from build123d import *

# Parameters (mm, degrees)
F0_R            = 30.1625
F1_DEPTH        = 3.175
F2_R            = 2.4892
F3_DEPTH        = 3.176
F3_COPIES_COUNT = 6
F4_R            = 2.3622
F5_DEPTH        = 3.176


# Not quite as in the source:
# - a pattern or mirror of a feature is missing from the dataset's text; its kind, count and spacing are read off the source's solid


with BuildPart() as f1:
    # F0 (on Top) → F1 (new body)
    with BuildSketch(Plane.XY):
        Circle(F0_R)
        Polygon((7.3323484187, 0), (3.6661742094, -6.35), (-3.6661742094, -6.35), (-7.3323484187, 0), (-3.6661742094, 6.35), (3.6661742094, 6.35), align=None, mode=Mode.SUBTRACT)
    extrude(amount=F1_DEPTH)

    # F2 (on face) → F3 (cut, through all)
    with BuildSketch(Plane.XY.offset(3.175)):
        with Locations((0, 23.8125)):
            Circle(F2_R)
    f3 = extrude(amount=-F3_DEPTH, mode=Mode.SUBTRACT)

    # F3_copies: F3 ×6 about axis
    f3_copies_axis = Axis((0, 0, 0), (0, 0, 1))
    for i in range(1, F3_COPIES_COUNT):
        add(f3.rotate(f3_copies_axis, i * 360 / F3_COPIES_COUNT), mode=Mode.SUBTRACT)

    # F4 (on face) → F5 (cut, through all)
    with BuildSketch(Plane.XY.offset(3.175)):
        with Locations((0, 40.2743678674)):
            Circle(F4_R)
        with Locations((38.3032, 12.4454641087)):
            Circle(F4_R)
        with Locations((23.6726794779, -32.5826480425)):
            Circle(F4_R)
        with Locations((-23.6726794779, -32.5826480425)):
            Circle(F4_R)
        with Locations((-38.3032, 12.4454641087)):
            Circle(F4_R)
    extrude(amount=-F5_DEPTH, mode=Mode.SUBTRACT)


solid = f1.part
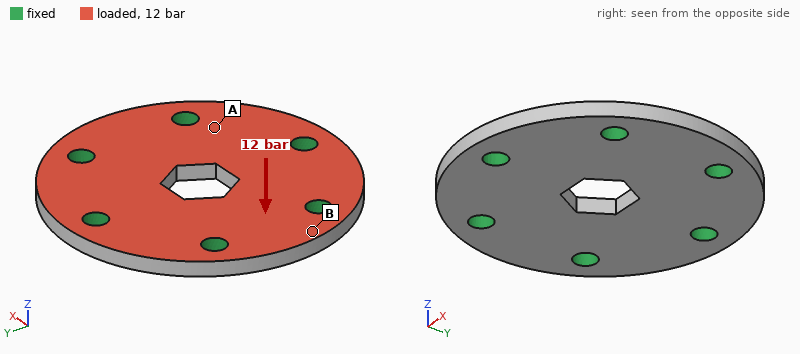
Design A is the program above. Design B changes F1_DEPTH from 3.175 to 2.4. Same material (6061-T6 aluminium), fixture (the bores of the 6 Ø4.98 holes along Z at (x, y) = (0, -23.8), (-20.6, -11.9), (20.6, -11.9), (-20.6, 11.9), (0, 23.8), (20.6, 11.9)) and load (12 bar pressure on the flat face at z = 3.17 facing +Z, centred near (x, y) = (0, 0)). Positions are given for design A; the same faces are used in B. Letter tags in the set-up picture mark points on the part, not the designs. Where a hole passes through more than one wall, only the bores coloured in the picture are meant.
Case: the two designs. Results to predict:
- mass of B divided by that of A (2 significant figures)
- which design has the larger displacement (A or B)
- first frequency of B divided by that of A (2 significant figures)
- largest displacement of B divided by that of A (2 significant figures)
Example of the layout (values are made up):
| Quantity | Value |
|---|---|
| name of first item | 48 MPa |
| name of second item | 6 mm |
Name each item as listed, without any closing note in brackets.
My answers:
| Quantity | Value |
|---|---|
| mass of B divided by that of A | 0.76 |
| which design has the larger displacement | B |
| first frequency of B divided by that of A | 0.79 |
| largest displacement of B divided by that of A | 2.2 |
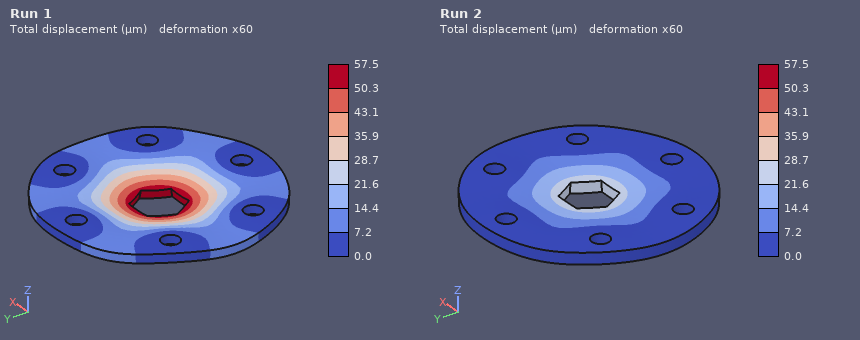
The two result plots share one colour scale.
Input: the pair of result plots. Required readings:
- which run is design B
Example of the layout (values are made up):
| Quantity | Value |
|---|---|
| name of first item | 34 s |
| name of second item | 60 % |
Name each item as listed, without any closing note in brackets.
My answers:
| Quantity | Value |
|---|---|
| which run is design B | Run 1 |
